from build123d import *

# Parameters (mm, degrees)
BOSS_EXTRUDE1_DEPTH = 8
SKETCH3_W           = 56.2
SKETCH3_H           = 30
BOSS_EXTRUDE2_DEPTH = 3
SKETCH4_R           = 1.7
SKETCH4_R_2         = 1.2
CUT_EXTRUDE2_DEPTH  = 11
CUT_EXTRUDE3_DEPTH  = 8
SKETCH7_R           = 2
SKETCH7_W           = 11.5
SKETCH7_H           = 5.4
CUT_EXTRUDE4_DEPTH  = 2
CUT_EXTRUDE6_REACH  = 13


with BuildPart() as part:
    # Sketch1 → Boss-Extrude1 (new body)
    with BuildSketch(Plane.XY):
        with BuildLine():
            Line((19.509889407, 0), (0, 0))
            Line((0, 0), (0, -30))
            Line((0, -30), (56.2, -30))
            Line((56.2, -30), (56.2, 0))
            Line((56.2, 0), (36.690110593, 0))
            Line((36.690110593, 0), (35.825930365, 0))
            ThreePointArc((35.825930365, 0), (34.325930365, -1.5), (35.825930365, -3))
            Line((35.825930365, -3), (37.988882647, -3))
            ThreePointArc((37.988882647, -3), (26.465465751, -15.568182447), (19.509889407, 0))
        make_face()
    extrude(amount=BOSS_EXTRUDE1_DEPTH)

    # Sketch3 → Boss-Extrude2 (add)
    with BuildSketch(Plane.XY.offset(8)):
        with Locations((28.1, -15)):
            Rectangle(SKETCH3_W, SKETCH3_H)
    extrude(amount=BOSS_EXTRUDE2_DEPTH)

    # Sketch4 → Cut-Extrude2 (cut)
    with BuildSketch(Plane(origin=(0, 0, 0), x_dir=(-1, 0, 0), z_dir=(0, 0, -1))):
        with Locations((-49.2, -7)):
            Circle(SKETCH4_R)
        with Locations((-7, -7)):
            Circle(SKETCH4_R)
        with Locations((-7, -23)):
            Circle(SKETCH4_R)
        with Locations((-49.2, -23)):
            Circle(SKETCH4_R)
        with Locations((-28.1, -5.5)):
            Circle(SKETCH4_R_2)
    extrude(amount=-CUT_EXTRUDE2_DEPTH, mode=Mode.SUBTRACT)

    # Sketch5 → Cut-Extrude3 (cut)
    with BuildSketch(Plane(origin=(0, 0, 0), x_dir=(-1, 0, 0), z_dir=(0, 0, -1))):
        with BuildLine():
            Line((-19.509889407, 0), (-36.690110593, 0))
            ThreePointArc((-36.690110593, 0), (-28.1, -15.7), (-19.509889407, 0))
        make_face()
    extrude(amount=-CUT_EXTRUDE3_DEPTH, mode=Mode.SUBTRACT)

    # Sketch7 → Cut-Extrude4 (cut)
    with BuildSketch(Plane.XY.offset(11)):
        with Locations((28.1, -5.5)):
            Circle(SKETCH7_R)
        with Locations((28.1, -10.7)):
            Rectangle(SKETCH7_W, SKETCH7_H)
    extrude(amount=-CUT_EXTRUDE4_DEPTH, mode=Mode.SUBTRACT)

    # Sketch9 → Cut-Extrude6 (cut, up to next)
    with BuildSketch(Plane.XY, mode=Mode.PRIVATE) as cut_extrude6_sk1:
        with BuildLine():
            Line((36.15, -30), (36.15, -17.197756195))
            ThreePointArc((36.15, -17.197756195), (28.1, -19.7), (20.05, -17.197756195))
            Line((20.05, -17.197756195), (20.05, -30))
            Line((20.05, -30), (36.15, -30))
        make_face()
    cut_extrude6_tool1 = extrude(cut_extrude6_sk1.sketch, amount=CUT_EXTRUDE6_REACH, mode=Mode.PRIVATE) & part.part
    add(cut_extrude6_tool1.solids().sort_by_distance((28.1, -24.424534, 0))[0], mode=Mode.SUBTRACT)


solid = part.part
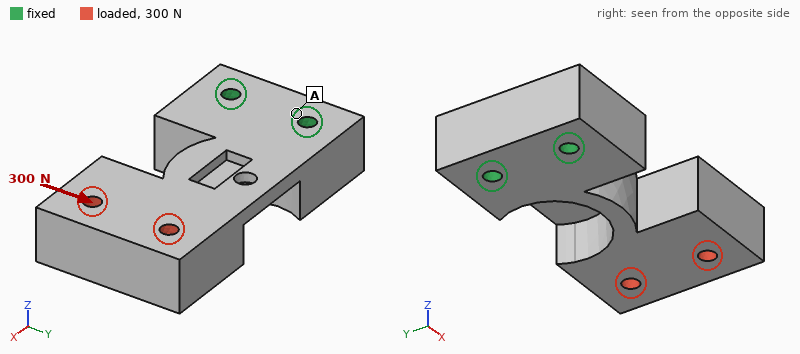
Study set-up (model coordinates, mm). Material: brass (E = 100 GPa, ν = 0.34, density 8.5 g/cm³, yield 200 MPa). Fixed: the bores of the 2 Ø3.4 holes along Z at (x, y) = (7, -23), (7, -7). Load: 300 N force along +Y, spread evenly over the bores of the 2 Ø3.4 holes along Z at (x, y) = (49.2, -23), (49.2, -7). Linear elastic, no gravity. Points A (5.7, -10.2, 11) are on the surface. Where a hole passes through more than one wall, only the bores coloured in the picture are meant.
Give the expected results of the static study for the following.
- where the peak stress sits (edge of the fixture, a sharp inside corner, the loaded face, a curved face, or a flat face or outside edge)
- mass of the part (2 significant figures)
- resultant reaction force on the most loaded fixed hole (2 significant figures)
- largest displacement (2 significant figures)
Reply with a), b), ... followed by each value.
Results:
a) a curved face
b) 120 g
c) 760 N
d) 58 µm
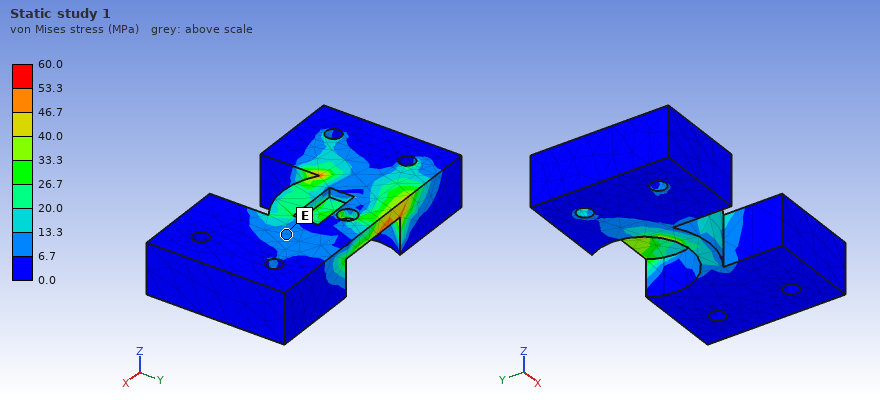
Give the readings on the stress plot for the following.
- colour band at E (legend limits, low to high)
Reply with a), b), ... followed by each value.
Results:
a) 6.7 to 13.3 MPa
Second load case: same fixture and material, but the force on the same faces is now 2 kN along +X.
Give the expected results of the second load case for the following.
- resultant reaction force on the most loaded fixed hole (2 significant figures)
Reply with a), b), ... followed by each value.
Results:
a) 1.1 kN
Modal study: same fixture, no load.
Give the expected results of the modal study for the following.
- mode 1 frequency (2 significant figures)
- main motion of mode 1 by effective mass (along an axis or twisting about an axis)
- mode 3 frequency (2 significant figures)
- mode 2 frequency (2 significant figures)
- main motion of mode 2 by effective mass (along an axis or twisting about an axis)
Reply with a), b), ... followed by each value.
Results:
a) 1300 Hz
b) along Z
c) 2800 Hz
d) 2100 Hz
e) along Y
